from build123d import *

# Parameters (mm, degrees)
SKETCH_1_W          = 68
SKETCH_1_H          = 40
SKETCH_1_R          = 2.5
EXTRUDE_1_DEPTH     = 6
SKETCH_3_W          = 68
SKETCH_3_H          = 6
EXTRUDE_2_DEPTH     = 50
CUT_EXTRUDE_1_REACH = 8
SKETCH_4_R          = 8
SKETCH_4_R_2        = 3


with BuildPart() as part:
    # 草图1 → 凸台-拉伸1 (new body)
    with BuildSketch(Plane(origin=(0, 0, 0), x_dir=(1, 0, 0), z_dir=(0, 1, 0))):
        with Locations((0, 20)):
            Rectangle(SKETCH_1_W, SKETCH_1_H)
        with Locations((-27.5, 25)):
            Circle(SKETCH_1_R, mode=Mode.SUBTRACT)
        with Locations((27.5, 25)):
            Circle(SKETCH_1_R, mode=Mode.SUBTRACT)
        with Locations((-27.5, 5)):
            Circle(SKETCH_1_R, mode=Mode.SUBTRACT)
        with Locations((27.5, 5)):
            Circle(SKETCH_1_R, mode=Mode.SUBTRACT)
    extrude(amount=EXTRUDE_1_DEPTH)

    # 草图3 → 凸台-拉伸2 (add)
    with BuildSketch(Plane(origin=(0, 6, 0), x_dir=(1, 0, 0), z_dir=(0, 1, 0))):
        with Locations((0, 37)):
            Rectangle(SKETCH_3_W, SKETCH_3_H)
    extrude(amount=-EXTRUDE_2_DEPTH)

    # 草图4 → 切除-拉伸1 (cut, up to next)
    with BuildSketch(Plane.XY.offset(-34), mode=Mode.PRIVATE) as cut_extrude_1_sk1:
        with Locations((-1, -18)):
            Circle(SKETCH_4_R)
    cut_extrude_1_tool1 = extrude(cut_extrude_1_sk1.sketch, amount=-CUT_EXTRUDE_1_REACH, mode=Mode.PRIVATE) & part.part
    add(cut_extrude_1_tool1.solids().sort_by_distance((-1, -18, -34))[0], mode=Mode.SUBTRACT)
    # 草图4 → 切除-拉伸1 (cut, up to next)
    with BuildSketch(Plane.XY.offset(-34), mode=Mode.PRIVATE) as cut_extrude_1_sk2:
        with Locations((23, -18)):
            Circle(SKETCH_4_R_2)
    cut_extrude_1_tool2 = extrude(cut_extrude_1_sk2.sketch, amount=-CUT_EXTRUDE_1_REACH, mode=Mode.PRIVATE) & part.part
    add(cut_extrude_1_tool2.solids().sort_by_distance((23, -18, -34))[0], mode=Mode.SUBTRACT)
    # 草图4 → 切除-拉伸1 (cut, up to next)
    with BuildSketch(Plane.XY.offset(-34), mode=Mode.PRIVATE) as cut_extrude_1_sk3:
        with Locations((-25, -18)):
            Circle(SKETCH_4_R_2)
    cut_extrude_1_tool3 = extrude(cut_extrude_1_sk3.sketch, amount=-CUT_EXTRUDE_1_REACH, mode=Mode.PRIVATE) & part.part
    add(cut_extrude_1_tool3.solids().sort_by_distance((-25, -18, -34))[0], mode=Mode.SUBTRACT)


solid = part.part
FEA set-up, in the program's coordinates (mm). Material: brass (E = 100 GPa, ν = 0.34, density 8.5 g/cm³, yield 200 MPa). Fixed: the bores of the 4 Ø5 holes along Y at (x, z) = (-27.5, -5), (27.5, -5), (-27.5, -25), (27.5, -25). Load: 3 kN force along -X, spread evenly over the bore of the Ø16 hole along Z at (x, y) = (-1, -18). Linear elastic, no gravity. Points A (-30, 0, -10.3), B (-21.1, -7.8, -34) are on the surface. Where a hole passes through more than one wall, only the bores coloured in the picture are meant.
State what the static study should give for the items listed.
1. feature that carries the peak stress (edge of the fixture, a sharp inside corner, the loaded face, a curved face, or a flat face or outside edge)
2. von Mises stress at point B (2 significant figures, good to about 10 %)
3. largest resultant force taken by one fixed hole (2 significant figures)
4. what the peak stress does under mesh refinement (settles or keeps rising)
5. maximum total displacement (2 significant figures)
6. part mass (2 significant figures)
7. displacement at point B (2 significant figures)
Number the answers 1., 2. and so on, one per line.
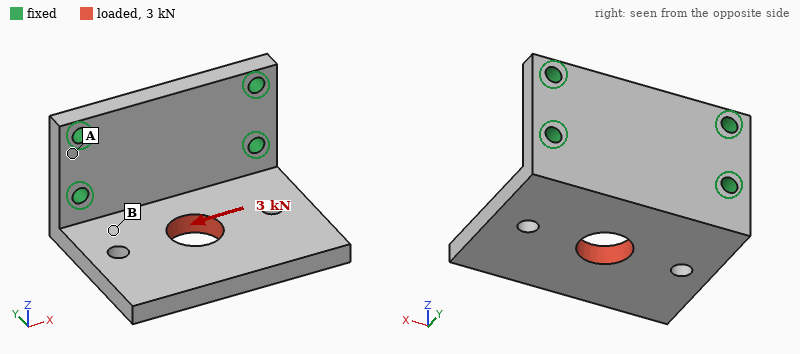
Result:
1. edge of the fixture
2. 27 MPa
3. 1.9 kN
4. keeps rising
5. 49 µm
6. 270 g
7. 16 µm
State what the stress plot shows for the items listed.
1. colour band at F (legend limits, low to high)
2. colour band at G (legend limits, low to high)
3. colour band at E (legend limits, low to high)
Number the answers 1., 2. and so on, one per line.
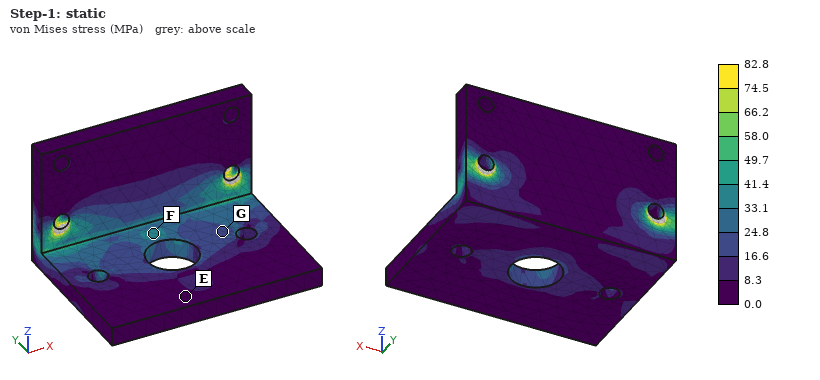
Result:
1. 33.1 to 41.4 MPa
2. 16.6 to 24.8 MPa
3. 0.0 to 8.3 MPa
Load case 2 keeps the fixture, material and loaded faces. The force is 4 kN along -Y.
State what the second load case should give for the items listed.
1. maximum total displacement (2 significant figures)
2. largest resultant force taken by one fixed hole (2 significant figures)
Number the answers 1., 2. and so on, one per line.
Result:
1. 0.15 mm
2. 2.5 kN
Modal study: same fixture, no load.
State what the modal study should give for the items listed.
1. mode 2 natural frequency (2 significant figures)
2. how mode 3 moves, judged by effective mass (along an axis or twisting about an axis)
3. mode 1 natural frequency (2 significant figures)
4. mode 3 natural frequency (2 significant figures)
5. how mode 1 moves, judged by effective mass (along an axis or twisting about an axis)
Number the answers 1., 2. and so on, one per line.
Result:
1. 2200 Hz
2. along X
3. 1100 Hz
4. 4100 Hz
5. along Z
